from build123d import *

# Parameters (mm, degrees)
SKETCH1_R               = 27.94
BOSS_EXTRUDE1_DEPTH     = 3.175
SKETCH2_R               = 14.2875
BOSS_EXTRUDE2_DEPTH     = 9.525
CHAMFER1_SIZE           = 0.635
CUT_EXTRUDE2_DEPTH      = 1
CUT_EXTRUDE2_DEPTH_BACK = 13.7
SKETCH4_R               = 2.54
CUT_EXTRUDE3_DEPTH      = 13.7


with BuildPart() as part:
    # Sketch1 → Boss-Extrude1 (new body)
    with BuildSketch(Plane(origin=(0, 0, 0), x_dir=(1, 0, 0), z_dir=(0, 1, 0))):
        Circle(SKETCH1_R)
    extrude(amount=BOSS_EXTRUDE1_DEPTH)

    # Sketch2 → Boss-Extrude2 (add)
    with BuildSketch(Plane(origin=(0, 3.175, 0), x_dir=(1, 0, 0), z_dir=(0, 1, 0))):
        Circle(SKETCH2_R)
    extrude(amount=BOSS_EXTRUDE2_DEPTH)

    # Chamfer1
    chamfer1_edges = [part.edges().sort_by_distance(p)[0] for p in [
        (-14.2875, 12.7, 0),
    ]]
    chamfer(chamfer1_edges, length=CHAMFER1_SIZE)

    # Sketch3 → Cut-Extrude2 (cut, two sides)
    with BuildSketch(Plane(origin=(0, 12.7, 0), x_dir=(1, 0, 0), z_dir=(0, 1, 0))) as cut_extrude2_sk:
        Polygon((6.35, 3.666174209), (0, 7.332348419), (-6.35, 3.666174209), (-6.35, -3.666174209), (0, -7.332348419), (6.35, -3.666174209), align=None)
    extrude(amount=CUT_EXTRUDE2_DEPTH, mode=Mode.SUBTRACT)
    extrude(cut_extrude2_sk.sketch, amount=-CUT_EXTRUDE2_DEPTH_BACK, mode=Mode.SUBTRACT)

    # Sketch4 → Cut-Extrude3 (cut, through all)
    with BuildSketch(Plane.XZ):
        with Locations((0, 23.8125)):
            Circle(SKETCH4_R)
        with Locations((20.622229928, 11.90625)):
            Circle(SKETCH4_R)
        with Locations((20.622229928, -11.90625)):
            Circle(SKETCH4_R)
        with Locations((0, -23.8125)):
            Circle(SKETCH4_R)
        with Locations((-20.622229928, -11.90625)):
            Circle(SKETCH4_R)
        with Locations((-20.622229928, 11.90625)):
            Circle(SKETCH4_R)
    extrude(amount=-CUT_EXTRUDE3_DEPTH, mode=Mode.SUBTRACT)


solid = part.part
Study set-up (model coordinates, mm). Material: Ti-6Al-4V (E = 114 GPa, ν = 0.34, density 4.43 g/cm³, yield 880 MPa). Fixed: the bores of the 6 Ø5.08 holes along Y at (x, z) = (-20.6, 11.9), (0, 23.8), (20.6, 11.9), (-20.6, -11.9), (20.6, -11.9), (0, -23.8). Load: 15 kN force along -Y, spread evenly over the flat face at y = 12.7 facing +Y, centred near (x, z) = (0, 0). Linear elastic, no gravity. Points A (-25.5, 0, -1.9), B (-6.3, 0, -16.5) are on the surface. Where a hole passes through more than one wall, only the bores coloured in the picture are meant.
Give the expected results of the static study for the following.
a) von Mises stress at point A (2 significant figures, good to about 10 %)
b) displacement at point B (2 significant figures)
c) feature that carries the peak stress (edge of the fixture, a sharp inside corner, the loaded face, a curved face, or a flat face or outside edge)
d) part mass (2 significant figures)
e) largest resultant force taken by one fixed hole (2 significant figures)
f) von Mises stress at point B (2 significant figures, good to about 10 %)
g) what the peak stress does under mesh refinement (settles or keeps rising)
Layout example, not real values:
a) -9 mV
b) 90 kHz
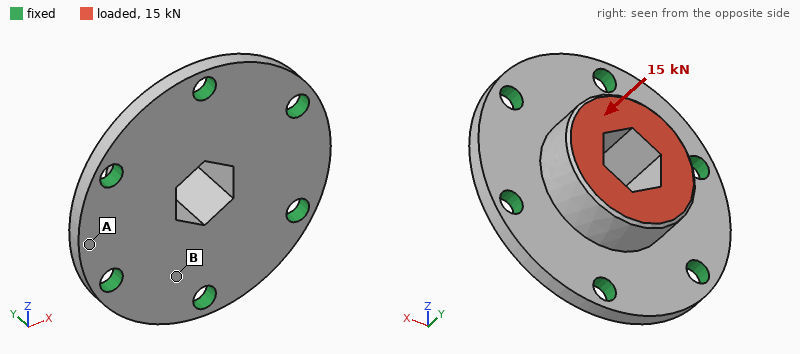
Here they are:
a) 51 MPa
b) 36 µm
c) edge of the fixture
d) 52 g
e) 2.9 kN
f) 110 MPa
g) keeps rising
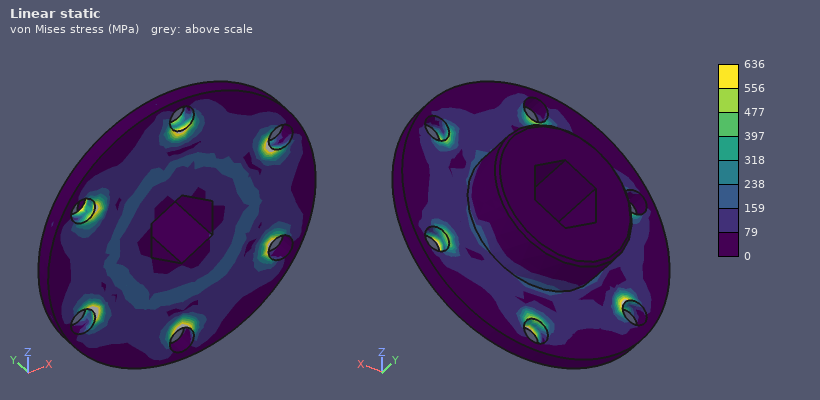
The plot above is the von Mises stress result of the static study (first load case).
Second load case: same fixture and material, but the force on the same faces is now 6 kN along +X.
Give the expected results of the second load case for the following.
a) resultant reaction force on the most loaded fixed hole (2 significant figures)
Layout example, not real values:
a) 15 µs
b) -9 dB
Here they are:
a) 1.6 kN
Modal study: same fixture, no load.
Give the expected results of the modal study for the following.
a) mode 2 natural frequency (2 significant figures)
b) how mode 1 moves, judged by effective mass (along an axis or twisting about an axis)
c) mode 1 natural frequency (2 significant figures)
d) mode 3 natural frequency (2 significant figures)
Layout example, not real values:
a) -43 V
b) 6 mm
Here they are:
a) 19 kHz
b) along Y
c) 14 kHz
d) 19 kHz
